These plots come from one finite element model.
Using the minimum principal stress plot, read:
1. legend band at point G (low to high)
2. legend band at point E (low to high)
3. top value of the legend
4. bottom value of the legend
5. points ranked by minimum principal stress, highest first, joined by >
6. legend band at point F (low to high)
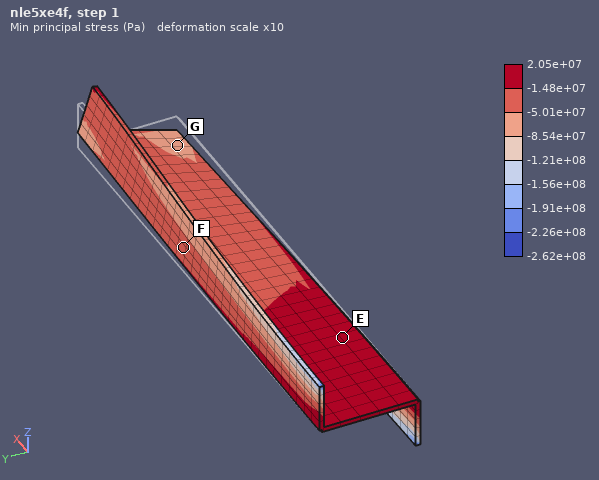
-8.54e+07 to -5.01e+07 Pa
-1.48e+07 to 2.05e+07 Pa
2.05e+07 Pa
-2.62e+08 Pa
E > F > G
-5.01e+07 to -1.48e+07 Pa
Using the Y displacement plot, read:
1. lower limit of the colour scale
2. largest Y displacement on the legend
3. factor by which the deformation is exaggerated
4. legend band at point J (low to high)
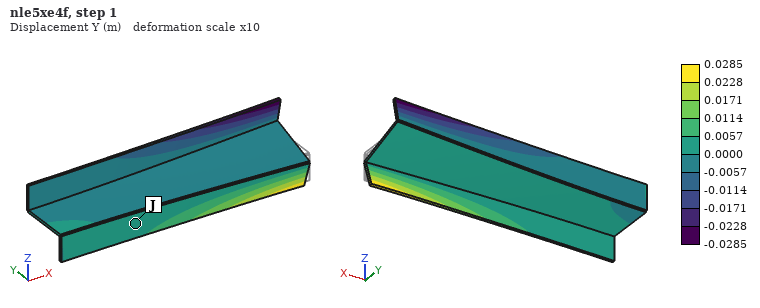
-0.0285 m
0.0285 m
10
0.0000 to 0.0057 m
